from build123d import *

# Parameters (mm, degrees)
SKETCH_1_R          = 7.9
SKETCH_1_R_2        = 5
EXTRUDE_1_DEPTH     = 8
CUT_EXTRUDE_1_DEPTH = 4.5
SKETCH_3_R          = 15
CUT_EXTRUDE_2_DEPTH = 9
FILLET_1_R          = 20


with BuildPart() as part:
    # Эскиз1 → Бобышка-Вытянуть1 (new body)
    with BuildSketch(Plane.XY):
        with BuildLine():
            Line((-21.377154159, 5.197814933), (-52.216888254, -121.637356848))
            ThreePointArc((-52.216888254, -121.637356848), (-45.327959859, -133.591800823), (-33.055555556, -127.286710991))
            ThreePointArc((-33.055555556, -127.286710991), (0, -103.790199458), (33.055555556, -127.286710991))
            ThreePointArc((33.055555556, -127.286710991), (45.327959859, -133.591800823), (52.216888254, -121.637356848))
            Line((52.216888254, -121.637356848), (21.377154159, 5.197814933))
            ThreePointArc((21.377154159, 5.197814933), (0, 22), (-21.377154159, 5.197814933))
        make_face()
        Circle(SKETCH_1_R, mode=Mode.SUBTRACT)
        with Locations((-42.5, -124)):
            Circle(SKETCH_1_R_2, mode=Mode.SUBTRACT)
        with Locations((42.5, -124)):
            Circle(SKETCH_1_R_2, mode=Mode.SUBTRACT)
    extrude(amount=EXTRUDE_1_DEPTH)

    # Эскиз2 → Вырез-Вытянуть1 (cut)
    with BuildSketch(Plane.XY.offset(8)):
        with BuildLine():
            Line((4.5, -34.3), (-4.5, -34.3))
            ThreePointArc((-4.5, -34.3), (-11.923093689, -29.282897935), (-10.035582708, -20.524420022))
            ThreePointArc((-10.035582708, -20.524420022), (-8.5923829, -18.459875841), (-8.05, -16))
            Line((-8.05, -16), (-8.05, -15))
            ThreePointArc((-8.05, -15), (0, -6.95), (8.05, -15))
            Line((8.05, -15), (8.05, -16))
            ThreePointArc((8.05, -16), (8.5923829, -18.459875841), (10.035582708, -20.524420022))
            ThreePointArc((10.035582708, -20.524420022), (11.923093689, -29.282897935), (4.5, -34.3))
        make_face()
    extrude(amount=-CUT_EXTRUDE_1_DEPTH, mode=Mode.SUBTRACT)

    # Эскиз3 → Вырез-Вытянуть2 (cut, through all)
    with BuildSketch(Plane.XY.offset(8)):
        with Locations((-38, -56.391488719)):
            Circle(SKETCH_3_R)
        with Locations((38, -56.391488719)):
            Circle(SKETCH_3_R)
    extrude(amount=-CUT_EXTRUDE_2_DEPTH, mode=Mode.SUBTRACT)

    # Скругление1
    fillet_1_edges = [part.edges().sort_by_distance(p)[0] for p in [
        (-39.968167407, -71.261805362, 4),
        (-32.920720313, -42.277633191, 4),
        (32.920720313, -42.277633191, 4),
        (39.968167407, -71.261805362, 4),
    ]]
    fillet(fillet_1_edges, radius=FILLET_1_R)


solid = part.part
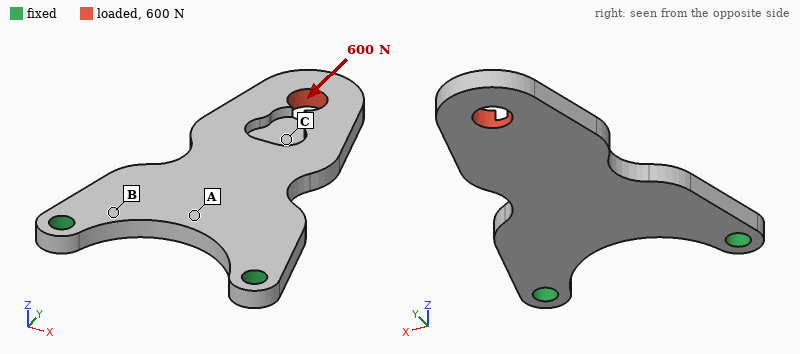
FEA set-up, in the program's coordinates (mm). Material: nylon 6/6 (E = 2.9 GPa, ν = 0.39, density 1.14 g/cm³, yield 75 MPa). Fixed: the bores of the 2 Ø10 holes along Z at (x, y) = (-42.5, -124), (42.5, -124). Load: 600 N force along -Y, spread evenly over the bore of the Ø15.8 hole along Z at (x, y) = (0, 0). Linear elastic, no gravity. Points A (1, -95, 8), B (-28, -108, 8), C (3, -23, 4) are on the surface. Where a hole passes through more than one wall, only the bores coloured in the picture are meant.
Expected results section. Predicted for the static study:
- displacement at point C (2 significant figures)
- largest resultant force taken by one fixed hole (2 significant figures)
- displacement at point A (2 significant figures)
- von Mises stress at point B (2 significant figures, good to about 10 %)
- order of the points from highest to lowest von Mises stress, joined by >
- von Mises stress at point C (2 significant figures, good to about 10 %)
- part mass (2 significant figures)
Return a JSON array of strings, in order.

["0.072 mm", "340 N", "0.032 mm", "1.6 MPa", "C > B > A", "3.1 MPa", "75 g"]
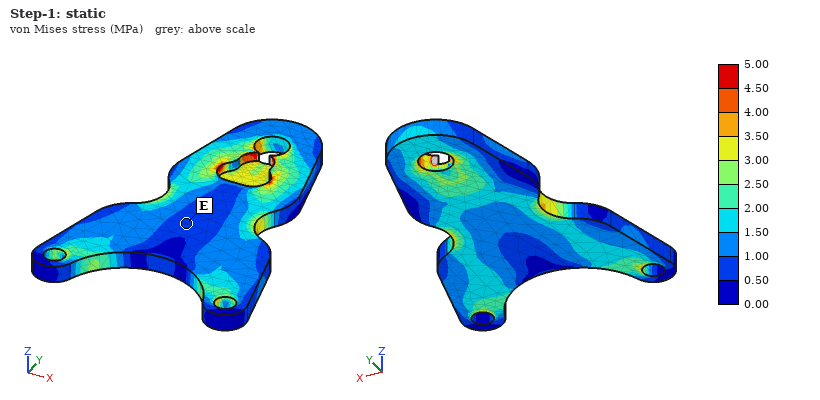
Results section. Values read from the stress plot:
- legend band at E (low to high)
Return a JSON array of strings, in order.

["0.50 to 1.00 MPa"]
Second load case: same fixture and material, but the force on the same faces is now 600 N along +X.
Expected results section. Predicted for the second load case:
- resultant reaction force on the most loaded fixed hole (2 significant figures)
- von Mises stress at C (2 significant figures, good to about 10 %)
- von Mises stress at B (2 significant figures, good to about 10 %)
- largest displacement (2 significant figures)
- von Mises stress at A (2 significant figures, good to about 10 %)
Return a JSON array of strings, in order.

["920 N", "7.9 MPa", "3.7 MPa", "1.0 mm", "1.8 MPa"]
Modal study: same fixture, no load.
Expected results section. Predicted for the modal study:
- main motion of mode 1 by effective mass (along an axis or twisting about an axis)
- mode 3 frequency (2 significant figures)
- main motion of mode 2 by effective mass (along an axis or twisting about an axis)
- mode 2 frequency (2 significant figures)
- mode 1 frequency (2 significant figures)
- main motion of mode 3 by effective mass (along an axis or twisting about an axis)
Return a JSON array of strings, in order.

["along Z", "630 Hz", "along Z", "600 Hz", "120 Hz", "twisting about Y"]
